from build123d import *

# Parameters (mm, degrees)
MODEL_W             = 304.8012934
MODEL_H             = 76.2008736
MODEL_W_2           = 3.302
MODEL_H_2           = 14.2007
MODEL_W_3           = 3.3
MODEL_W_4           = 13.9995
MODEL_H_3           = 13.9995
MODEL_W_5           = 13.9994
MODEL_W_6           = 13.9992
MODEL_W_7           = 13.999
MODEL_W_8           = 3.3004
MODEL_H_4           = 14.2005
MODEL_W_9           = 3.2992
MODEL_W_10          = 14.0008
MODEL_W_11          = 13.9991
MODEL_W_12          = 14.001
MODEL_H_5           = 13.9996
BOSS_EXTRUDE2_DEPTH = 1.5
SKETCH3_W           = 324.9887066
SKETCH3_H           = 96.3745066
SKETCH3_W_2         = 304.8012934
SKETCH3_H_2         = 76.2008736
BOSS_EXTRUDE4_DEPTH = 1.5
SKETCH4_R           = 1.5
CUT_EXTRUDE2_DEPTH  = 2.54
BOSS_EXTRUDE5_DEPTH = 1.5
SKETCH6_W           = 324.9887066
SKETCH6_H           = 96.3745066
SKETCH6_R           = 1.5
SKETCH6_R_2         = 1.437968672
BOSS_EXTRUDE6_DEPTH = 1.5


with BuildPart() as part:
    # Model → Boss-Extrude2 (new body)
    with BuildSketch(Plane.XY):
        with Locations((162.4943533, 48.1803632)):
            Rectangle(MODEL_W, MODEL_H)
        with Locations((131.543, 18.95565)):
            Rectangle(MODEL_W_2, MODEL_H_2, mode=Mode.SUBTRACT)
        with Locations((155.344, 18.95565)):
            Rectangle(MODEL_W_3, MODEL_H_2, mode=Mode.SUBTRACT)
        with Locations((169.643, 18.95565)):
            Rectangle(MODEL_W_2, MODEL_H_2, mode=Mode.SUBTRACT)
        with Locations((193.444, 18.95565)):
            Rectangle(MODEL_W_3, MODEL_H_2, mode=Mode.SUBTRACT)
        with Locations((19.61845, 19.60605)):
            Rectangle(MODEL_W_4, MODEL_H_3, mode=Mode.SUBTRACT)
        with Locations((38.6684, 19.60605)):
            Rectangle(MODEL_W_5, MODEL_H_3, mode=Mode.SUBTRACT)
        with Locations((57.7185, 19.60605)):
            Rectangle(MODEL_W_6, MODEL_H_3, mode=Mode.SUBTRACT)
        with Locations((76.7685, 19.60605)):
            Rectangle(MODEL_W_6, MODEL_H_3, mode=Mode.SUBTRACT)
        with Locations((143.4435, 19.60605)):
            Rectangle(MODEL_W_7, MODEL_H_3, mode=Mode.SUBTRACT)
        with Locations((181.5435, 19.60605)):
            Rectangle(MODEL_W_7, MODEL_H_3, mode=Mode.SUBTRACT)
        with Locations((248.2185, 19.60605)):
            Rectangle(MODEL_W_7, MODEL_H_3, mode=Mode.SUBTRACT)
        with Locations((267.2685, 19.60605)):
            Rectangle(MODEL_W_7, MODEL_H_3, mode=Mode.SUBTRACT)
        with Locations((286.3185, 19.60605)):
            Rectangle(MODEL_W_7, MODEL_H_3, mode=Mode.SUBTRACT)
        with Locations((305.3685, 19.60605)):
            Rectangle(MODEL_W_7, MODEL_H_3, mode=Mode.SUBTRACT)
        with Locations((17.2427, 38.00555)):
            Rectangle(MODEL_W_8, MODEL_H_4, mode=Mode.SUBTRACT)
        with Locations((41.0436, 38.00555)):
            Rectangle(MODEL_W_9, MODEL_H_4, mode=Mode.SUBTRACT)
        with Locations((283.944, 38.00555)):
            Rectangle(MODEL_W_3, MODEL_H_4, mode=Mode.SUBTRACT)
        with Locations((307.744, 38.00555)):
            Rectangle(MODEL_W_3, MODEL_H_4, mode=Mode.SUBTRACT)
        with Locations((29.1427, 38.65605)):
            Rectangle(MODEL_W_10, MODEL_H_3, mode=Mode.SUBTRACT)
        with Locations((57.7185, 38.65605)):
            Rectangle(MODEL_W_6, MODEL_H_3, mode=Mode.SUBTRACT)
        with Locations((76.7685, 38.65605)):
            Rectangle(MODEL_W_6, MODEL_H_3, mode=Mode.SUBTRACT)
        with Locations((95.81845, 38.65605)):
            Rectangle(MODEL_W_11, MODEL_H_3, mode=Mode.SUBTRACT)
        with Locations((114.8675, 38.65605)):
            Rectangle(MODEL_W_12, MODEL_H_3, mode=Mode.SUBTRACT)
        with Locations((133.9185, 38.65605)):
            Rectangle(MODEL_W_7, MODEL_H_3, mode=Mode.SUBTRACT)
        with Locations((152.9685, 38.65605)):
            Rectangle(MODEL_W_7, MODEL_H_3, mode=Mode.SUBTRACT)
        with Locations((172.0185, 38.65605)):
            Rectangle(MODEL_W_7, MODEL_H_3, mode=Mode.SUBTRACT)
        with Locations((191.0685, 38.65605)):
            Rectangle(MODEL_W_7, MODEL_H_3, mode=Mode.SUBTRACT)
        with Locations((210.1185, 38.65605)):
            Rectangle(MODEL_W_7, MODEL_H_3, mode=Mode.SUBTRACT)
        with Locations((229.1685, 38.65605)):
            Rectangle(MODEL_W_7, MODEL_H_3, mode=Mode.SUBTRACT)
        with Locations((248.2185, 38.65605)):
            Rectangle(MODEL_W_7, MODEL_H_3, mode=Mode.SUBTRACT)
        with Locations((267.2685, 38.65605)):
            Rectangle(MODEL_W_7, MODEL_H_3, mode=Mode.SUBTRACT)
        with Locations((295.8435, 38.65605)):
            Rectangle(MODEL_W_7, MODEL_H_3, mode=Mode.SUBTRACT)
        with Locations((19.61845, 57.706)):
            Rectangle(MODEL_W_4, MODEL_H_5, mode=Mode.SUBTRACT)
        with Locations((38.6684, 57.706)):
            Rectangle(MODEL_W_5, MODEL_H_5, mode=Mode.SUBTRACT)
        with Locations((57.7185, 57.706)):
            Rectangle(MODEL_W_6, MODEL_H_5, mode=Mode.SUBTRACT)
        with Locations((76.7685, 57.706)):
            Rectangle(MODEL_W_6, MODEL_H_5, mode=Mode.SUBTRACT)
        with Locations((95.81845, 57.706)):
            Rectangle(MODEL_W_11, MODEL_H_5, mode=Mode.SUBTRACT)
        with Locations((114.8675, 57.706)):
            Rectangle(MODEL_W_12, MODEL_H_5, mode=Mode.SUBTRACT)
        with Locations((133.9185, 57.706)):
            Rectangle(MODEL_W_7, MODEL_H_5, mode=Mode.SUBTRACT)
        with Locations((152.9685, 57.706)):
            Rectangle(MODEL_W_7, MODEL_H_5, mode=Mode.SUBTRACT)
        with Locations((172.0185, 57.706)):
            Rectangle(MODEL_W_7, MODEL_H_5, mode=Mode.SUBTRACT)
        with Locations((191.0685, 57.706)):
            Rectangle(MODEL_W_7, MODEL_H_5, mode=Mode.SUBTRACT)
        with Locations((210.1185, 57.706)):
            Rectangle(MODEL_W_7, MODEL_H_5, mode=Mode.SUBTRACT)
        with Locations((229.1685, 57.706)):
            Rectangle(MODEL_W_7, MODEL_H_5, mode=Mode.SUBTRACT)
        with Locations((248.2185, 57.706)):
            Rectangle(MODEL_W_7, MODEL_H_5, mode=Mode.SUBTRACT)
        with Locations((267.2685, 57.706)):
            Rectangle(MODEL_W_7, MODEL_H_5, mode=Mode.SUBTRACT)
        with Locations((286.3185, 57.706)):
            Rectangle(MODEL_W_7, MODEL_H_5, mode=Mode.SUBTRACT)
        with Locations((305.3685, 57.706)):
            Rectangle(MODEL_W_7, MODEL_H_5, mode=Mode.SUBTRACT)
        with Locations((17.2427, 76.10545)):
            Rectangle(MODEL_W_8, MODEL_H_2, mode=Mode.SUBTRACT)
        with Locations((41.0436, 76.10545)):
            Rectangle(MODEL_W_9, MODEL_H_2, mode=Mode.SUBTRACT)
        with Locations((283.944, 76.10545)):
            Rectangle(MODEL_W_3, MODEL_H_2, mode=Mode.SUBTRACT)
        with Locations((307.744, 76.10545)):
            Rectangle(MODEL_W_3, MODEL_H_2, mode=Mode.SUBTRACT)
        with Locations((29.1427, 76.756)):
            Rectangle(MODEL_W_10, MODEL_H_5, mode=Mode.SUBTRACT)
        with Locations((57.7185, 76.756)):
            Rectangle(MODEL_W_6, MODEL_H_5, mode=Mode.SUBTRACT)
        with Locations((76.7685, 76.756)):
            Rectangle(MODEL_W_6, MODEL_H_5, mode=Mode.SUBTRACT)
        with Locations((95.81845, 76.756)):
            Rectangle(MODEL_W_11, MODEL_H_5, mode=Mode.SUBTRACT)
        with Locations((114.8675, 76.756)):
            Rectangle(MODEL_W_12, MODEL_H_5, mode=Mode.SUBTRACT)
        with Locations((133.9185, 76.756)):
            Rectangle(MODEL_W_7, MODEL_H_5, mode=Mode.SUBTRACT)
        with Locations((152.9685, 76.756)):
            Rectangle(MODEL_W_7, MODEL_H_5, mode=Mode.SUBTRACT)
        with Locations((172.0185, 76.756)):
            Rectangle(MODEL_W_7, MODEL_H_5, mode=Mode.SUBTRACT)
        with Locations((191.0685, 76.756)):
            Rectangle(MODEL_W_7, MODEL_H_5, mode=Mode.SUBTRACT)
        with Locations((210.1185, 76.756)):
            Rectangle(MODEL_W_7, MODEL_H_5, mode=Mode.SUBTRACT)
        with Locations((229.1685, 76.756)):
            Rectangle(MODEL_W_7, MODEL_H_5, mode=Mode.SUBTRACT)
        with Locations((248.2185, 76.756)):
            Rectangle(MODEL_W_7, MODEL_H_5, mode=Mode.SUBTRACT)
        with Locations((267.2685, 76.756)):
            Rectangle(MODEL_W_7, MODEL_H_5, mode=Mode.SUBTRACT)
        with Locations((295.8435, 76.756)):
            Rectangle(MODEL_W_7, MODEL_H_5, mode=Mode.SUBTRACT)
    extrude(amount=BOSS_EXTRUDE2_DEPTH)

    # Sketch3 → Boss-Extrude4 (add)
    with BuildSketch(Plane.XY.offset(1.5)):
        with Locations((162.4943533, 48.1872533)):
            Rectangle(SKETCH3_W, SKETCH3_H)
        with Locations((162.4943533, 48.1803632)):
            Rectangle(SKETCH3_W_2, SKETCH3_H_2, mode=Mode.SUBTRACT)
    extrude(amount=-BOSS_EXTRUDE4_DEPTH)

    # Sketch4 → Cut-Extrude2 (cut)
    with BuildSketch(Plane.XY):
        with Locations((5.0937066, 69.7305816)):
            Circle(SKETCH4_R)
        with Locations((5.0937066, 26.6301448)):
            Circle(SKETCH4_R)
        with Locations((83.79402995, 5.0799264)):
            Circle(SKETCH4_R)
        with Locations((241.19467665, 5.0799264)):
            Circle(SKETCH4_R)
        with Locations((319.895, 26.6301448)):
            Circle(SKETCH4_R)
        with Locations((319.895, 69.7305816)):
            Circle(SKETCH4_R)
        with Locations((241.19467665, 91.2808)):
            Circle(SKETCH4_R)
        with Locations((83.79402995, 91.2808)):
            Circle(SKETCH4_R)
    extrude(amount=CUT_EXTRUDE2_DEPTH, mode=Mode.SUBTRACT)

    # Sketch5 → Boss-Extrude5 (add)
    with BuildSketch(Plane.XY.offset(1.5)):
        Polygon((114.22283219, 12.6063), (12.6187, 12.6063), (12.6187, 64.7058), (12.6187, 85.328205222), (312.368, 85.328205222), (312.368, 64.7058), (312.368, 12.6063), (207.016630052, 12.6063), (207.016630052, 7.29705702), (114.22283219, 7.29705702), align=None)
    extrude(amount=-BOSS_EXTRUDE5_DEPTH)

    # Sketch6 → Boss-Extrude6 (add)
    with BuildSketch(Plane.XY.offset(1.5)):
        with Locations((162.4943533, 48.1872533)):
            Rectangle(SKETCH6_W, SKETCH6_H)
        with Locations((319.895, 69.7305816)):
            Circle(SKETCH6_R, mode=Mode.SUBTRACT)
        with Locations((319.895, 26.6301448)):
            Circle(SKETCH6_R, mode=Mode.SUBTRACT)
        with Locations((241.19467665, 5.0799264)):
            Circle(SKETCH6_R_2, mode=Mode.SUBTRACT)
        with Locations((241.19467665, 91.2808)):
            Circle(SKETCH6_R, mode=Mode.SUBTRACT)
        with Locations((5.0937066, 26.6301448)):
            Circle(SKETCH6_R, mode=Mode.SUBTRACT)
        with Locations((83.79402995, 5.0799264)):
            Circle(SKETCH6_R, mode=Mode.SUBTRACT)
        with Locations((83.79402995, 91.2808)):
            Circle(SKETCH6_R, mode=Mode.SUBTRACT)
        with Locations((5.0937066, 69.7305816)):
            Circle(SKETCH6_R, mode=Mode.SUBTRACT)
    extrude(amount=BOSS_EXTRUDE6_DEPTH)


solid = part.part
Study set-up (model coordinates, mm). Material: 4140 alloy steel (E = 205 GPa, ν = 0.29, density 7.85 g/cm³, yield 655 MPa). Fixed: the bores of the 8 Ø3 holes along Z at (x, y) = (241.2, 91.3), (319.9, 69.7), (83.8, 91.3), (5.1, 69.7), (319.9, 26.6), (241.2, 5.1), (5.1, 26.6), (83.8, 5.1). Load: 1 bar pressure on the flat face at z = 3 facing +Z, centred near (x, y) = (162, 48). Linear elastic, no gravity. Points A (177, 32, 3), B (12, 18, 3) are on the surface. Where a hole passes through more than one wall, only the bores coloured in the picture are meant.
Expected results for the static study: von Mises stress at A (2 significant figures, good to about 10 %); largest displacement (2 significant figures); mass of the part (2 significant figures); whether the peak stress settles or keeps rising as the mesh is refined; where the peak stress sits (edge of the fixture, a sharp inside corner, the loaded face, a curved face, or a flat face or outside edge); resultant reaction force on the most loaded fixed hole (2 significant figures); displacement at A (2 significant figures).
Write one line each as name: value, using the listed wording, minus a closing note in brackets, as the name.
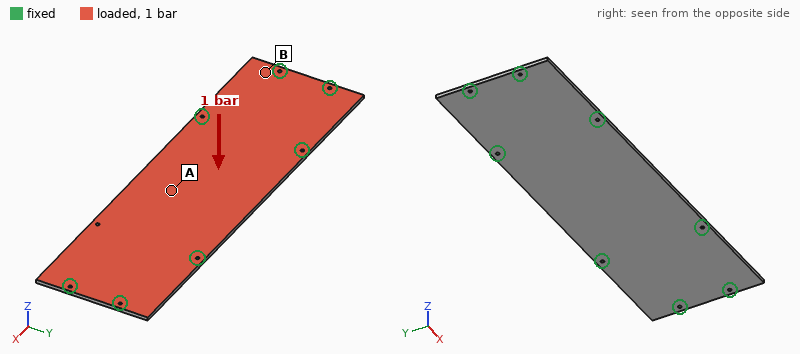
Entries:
von Mises stress at A: 66 MPa
largest displacement: 0.48 mm
mass of the part: 740 g
whether the peak stress settles or keeps rising as the mesh is refined: keeps rising
where the peak stress sits: edge of the fixture
resultant reaction force on the most loaded fixed hole: 690 N
displacement at A: 0.46 mm
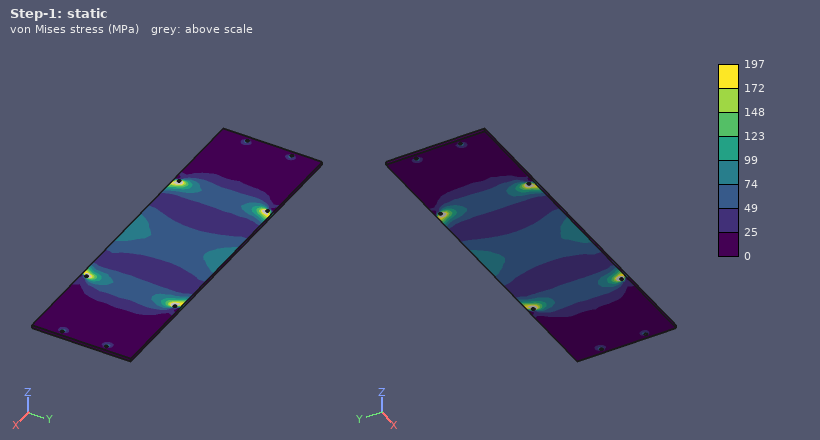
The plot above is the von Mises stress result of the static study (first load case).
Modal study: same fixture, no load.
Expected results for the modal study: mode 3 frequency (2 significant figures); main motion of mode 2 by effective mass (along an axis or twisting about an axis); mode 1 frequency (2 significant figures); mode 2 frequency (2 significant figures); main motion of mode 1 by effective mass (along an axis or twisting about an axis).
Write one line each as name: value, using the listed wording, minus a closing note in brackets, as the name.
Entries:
mode 3 frequency: 1400 Hz
main motion of mode 2 by effective mass: twisting about X
mode 1 frequency: 530 Hz
mode 2 frequency: 910 Hz
main motion of mode 1 by effective mass: along Z
